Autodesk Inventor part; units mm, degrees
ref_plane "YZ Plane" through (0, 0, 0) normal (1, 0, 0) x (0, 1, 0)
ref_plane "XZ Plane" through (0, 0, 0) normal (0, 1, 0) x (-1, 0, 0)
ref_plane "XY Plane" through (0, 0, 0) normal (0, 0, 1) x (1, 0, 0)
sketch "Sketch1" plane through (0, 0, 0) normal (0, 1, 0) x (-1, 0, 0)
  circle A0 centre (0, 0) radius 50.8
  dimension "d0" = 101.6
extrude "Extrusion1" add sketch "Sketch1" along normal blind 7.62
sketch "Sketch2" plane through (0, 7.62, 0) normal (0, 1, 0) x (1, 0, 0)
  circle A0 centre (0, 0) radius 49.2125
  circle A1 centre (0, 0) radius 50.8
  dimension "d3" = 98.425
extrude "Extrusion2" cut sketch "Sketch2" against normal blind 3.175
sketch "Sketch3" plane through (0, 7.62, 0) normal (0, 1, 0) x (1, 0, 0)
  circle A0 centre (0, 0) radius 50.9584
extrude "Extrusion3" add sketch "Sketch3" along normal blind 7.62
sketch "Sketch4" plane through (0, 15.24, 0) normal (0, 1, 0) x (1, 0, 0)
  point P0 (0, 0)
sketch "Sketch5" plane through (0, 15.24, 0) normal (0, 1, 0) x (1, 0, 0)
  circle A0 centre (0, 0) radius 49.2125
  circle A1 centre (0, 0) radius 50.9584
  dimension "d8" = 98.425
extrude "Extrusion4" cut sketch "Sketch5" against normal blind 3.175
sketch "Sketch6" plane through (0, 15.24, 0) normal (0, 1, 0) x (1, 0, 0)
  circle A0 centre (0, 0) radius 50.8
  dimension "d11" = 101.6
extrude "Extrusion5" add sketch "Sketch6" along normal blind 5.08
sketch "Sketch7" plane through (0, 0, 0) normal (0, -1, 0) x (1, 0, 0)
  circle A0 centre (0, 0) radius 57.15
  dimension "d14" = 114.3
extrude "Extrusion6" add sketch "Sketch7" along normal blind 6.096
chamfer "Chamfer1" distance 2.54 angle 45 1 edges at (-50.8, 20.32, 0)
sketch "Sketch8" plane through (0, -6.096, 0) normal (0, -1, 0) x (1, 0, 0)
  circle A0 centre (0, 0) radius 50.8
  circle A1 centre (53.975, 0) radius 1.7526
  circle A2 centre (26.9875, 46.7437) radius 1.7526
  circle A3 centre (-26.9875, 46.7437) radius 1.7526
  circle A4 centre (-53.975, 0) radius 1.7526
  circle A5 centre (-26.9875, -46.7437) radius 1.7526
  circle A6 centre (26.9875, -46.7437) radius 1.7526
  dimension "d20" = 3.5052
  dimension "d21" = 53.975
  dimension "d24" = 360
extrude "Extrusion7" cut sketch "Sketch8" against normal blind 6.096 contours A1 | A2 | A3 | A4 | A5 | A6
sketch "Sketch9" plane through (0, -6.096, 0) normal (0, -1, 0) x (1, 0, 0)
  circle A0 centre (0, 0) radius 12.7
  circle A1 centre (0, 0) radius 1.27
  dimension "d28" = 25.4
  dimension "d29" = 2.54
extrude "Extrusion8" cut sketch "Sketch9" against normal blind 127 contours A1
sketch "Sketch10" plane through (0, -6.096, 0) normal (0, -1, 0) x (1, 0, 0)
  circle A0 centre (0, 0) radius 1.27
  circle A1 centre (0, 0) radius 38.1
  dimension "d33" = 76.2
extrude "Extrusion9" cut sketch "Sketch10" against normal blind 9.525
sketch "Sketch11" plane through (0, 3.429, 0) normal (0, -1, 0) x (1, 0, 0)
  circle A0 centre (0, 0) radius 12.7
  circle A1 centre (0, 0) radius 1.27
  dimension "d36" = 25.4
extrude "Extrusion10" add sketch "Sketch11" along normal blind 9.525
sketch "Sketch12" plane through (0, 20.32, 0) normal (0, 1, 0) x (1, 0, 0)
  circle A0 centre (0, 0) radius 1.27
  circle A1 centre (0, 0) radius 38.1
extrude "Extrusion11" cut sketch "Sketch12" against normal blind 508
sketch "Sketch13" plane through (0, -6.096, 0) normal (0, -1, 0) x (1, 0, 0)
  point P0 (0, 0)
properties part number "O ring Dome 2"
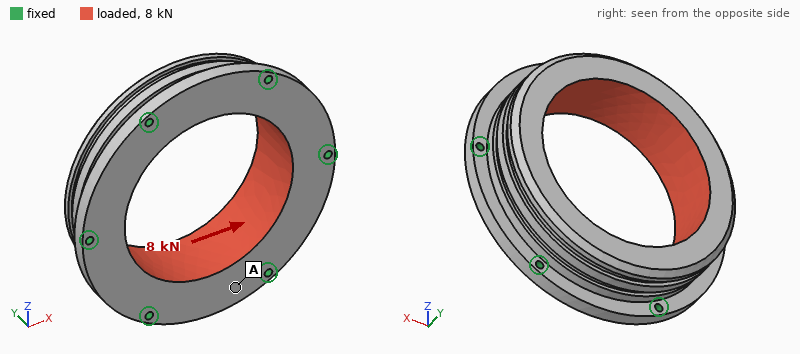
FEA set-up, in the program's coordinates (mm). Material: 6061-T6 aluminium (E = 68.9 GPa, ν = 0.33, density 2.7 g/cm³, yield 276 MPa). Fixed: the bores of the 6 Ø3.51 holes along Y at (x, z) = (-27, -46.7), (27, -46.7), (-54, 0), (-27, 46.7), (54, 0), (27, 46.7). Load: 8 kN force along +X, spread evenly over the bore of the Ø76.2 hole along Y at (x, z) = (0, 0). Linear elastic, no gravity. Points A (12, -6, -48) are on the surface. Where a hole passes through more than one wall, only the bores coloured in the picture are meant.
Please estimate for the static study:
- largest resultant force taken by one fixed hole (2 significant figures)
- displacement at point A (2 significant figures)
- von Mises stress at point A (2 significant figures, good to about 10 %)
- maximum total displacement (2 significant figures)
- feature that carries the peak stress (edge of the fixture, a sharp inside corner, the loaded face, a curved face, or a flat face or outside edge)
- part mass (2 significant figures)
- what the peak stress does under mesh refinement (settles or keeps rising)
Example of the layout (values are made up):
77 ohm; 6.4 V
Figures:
1.4 kN; 2.3 µm; 6.7 MPa; 7.9 µm; edge of the fixture; 280 g; keeps rising
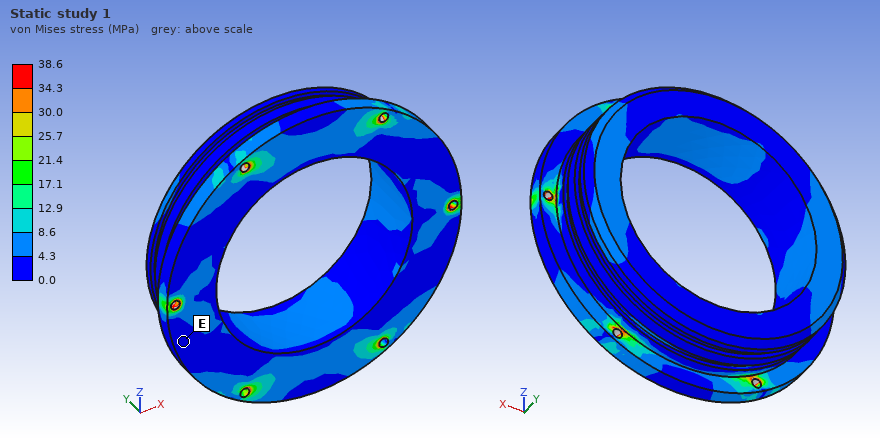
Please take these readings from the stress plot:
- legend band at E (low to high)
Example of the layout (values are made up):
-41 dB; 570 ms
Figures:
0.0 to 4.3 MPa
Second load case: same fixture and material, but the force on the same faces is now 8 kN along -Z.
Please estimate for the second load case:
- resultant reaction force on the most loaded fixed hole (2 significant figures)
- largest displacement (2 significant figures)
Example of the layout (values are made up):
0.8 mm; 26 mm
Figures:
1.4 kN; 8.6 µm
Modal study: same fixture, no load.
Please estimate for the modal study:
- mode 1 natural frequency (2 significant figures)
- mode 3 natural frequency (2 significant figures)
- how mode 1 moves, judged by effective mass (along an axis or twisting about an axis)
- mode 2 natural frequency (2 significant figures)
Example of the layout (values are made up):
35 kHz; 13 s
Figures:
10 kHz; 11 kHz; along Y; 11 kHz
